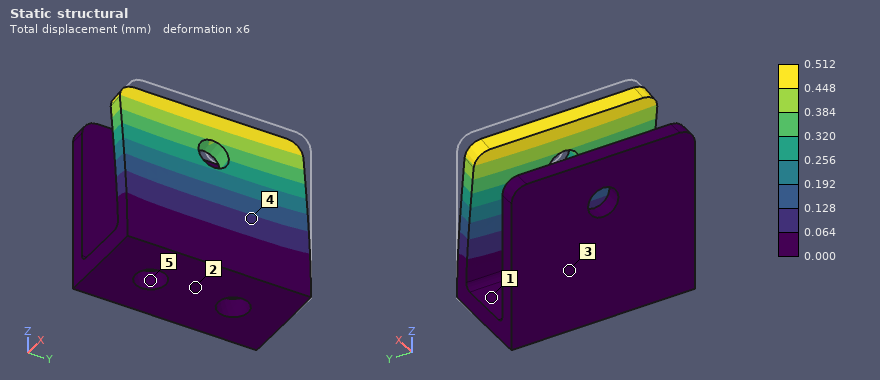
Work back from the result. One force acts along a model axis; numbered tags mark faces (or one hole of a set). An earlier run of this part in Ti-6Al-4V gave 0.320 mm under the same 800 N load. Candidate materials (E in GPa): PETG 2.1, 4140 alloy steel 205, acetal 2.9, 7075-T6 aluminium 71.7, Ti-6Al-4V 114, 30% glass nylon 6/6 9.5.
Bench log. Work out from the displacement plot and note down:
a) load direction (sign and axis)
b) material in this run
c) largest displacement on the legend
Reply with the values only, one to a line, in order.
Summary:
-X
7075-T6 aluminium
0.512 mm
